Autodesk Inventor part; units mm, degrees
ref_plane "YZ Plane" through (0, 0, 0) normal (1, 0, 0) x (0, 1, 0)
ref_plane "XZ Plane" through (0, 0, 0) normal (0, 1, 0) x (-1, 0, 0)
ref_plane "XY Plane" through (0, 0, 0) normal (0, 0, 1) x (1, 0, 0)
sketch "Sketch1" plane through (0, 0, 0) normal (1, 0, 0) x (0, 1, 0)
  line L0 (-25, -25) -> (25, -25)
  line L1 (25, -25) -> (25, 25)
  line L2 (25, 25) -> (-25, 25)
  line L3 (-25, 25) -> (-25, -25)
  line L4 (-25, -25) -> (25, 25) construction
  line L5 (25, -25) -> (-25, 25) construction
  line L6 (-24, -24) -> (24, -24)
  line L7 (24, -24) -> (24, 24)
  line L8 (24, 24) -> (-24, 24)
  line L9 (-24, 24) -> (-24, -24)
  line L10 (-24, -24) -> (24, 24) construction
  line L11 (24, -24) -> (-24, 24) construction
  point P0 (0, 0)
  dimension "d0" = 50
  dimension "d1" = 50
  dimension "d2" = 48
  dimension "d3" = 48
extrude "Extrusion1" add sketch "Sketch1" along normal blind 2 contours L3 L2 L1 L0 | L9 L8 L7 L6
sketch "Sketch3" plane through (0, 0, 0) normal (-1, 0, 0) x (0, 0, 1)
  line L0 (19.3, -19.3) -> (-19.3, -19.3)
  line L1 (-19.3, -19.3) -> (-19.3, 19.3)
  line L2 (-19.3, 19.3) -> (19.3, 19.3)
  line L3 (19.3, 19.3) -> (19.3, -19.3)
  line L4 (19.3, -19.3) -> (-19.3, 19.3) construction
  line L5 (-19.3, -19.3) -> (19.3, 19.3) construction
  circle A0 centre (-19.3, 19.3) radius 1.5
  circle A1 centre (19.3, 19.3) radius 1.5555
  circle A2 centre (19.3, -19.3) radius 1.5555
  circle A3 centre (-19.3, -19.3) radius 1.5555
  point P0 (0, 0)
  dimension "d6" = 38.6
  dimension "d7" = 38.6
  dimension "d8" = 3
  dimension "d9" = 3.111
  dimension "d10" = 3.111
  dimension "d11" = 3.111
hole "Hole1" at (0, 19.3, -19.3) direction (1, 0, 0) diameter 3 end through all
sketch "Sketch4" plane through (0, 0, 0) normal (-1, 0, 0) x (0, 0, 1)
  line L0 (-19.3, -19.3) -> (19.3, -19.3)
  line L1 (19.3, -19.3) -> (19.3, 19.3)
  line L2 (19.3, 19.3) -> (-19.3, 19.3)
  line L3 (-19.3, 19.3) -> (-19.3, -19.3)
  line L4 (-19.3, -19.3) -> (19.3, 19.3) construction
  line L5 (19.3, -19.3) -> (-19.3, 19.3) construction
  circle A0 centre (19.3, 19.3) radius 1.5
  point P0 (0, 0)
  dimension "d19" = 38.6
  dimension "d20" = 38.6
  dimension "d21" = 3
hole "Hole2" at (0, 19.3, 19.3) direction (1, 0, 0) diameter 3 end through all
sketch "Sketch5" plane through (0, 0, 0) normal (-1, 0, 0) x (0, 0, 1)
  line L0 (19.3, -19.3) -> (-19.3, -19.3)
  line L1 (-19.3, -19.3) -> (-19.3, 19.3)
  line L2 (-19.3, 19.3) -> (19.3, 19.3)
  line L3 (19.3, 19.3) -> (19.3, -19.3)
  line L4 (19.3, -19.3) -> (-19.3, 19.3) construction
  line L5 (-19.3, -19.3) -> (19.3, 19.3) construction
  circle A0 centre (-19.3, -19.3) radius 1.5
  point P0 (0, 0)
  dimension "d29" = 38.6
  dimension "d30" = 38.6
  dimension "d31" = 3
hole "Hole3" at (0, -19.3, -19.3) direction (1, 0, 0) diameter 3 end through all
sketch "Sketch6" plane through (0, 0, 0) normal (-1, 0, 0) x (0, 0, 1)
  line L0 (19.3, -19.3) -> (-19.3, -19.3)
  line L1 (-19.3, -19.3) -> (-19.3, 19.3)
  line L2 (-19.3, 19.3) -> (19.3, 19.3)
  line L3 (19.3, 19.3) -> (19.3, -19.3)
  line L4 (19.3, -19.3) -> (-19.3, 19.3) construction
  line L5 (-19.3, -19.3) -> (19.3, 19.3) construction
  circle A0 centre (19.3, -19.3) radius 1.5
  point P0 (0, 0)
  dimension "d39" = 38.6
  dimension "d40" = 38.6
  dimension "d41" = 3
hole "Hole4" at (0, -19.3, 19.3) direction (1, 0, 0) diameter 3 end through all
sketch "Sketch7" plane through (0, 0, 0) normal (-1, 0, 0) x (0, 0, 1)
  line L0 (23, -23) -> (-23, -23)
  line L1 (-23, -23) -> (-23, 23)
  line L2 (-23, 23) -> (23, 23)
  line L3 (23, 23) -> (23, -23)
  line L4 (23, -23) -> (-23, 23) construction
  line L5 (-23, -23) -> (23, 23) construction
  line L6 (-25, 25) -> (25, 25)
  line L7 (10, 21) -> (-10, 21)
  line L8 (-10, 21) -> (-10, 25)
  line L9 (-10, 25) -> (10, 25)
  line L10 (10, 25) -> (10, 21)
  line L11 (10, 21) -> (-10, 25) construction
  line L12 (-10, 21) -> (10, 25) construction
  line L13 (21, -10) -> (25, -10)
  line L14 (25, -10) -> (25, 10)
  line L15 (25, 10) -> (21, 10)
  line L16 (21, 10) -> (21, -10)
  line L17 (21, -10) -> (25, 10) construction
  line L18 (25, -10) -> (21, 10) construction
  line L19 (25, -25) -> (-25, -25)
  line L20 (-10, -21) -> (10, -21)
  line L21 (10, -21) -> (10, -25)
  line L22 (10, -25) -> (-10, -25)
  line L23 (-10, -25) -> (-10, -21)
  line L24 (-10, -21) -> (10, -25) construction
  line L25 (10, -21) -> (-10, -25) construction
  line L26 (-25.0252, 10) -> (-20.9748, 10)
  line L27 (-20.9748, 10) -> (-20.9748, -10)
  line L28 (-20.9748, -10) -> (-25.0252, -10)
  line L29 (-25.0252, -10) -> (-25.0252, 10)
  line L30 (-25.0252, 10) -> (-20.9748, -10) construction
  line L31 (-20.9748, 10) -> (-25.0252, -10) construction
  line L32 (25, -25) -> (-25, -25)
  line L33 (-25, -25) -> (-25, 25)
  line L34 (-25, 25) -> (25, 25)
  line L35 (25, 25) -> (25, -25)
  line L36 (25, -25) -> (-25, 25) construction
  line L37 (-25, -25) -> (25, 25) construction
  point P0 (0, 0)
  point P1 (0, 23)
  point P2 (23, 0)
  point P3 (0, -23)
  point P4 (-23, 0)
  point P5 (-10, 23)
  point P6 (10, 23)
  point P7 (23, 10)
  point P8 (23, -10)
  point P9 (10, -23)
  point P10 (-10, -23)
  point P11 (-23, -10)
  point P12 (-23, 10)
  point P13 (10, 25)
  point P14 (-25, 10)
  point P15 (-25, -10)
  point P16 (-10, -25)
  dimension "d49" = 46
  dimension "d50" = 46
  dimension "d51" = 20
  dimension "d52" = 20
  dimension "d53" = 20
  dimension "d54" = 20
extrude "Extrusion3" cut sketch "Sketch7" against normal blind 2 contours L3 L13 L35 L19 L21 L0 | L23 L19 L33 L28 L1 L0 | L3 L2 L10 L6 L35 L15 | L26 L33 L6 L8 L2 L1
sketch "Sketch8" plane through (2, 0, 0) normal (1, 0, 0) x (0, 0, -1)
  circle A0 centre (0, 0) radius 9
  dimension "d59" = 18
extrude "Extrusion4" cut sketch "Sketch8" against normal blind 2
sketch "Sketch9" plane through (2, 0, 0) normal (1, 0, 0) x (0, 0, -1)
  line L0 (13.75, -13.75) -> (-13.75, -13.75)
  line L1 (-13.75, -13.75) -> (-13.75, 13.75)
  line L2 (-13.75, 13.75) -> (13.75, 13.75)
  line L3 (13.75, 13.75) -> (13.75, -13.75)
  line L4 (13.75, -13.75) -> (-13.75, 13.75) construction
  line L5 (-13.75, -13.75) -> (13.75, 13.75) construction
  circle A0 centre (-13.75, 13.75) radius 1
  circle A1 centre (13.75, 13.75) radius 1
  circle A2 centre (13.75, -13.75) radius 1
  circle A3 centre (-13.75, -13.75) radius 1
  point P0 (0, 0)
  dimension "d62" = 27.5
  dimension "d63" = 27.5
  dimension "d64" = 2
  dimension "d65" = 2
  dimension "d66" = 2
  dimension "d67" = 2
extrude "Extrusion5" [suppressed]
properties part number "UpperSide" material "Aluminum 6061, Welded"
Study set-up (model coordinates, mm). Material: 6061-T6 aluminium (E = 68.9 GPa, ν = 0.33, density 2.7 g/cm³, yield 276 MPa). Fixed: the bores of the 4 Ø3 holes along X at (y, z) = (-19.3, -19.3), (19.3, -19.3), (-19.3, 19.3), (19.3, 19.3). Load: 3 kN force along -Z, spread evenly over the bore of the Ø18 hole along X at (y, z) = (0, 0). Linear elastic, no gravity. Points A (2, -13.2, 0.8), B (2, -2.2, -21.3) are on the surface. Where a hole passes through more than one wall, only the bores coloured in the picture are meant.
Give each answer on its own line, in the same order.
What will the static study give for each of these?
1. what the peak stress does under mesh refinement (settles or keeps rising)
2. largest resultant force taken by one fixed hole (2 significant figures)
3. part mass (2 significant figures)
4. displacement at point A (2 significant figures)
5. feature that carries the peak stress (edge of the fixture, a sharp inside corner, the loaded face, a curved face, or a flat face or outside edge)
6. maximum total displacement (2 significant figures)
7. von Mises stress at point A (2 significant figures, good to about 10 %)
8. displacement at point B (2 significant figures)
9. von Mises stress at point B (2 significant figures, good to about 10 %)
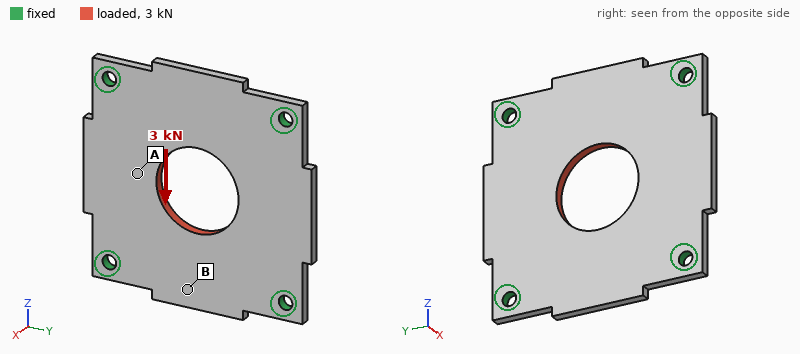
keeps rising
810 N
11 g
8.3 µm
edge of the fixture
15 µm
34 MPa
12 µm
15 MPa
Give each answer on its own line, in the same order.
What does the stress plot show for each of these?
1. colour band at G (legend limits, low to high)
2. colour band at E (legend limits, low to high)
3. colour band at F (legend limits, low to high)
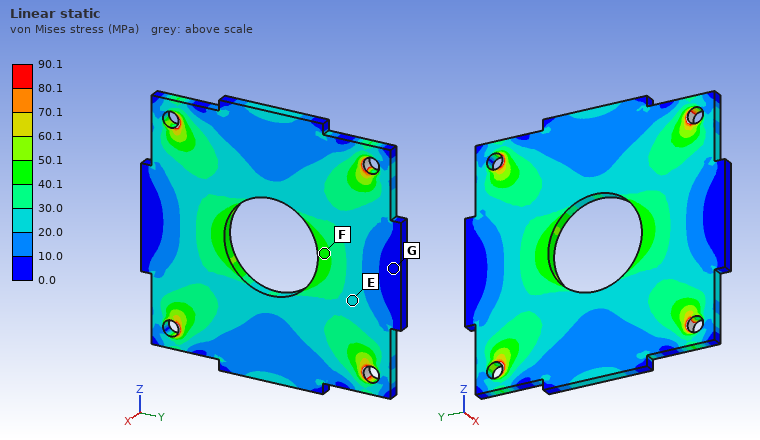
0.0 to 10.0 MPa
20.0 to 30.0 MPa
40.1 to 50.1 MPa
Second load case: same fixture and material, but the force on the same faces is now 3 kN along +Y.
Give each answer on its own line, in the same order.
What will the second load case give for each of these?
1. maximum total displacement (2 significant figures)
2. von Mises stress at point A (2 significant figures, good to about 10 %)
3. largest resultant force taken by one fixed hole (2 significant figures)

15 µm
18 MPa
810 N
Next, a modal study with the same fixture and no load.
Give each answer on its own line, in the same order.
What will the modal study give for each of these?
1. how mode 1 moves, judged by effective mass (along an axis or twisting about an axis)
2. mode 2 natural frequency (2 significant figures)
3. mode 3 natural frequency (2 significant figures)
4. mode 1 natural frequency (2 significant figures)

along X
7300 Hz
7300 Hz
5200 Hz
